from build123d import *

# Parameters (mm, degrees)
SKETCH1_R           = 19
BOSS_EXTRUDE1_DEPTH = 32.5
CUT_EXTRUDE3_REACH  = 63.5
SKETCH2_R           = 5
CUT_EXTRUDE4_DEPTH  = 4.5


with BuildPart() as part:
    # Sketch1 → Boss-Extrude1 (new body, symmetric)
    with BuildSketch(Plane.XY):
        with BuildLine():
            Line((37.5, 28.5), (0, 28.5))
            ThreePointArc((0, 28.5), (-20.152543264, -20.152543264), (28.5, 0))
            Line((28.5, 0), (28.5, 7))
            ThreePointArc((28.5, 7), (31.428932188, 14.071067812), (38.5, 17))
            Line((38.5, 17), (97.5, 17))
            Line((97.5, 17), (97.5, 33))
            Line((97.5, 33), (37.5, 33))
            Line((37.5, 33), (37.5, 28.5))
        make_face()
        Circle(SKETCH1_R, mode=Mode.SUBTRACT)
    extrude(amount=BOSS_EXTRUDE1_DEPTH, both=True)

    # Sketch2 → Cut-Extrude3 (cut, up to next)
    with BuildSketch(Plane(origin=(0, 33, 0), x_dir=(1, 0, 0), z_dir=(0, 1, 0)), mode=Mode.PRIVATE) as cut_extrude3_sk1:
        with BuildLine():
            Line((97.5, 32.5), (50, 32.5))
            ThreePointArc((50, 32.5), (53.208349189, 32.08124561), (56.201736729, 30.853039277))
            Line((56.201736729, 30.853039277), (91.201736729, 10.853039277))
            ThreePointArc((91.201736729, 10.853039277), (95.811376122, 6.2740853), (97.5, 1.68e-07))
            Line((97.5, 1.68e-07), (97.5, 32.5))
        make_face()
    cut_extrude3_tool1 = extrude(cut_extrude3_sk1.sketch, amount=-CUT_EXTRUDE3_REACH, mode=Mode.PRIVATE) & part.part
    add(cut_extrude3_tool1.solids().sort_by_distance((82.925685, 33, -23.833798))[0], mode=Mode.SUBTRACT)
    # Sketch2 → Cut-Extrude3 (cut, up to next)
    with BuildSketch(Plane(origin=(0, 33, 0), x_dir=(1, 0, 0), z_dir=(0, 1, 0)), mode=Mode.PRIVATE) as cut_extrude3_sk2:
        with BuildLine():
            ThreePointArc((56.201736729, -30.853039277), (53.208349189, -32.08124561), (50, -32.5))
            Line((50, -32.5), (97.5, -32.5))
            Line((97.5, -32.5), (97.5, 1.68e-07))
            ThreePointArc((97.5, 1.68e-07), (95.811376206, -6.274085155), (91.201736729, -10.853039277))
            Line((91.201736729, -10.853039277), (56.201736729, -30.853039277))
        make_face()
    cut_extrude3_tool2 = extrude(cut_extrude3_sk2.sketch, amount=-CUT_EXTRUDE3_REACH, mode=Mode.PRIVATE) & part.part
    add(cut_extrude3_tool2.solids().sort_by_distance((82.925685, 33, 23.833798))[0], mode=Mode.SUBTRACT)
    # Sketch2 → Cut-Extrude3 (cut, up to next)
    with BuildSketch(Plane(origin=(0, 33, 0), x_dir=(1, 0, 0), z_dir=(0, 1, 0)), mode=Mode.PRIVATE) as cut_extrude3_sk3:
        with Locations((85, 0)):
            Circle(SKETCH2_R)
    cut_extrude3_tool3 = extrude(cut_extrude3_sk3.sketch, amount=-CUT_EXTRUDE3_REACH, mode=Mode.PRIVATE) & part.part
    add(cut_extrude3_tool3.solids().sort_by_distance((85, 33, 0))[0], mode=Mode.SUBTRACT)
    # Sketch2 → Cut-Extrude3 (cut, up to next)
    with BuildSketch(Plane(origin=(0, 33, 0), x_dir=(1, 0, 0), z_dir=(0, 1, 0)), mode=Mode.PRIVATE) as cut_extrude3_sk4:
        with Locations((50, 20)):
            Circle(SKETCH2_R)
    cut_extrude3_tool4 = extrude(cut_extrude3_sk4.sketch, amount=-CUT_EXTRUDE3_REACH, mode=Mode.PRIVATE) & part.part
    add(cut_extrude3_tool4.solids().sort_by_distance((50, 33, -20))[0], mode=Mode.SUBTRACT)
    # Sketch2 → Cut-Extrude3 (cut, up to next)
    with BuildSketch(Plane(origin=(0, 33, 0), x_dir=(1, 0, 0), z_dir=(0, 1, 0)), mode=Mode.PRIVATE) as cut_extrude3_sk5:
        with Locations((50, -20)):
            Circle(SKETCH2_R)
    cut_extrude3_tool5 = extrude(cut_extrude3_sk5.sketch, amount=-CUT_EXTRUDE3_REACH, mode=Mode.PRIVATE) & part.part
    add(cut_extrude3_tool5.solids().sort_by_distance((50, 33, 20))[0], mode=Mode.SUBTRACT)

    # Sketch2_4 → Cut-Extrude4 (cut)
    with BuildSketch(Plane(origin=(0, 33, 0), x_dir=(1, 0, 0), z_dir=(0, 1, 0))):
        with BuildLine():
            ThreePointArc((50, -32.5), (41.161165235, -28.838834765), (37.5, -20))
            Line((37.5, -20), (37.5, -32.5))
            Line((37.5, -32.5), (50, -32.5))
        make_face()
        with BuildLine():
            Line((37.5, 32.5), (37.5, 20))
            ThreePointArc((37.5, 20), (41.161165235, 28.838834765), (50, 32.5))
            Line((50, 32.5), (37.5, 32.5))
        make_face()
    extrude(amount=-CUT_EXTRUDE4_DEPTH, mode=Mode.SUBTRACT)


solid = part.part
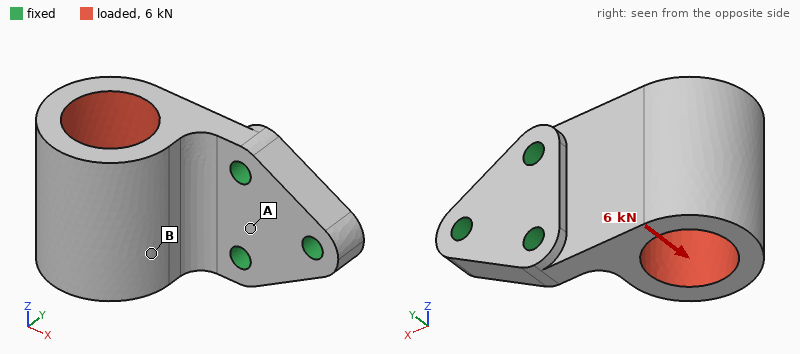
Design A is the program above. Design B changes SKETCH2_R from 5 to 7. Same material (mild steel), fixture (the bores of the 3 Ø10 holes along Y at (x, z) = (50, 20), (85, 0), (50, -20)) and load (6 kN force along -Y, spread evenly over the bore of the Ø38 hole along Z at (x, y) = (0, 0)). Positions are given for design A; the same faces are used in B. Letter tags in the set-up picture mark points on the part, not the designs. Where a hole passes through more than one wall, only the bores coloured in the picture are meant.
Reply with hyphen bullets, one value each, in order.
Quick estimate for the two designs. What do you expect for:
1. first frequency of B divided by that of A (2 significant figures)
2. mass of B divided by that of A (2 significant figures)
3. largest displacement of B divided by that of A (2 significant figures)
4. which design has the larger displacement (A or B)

- 1.0
- 0.98
- 0.91
- A
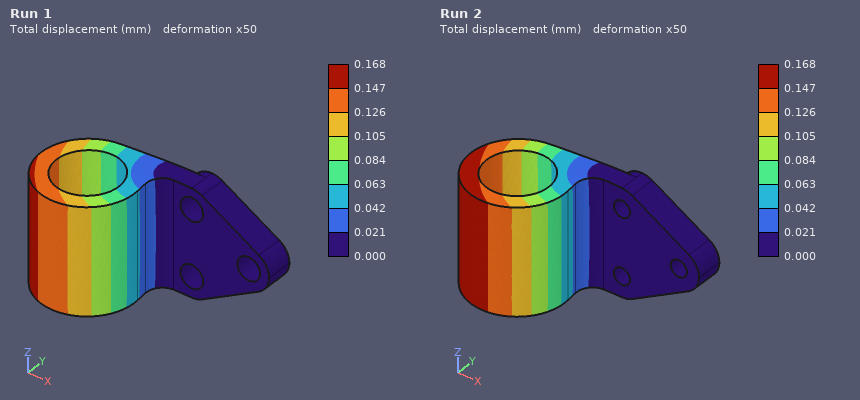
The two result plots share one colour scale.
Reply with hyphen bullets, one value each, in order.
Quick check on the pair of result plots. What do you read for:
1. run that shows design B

- Run 1
